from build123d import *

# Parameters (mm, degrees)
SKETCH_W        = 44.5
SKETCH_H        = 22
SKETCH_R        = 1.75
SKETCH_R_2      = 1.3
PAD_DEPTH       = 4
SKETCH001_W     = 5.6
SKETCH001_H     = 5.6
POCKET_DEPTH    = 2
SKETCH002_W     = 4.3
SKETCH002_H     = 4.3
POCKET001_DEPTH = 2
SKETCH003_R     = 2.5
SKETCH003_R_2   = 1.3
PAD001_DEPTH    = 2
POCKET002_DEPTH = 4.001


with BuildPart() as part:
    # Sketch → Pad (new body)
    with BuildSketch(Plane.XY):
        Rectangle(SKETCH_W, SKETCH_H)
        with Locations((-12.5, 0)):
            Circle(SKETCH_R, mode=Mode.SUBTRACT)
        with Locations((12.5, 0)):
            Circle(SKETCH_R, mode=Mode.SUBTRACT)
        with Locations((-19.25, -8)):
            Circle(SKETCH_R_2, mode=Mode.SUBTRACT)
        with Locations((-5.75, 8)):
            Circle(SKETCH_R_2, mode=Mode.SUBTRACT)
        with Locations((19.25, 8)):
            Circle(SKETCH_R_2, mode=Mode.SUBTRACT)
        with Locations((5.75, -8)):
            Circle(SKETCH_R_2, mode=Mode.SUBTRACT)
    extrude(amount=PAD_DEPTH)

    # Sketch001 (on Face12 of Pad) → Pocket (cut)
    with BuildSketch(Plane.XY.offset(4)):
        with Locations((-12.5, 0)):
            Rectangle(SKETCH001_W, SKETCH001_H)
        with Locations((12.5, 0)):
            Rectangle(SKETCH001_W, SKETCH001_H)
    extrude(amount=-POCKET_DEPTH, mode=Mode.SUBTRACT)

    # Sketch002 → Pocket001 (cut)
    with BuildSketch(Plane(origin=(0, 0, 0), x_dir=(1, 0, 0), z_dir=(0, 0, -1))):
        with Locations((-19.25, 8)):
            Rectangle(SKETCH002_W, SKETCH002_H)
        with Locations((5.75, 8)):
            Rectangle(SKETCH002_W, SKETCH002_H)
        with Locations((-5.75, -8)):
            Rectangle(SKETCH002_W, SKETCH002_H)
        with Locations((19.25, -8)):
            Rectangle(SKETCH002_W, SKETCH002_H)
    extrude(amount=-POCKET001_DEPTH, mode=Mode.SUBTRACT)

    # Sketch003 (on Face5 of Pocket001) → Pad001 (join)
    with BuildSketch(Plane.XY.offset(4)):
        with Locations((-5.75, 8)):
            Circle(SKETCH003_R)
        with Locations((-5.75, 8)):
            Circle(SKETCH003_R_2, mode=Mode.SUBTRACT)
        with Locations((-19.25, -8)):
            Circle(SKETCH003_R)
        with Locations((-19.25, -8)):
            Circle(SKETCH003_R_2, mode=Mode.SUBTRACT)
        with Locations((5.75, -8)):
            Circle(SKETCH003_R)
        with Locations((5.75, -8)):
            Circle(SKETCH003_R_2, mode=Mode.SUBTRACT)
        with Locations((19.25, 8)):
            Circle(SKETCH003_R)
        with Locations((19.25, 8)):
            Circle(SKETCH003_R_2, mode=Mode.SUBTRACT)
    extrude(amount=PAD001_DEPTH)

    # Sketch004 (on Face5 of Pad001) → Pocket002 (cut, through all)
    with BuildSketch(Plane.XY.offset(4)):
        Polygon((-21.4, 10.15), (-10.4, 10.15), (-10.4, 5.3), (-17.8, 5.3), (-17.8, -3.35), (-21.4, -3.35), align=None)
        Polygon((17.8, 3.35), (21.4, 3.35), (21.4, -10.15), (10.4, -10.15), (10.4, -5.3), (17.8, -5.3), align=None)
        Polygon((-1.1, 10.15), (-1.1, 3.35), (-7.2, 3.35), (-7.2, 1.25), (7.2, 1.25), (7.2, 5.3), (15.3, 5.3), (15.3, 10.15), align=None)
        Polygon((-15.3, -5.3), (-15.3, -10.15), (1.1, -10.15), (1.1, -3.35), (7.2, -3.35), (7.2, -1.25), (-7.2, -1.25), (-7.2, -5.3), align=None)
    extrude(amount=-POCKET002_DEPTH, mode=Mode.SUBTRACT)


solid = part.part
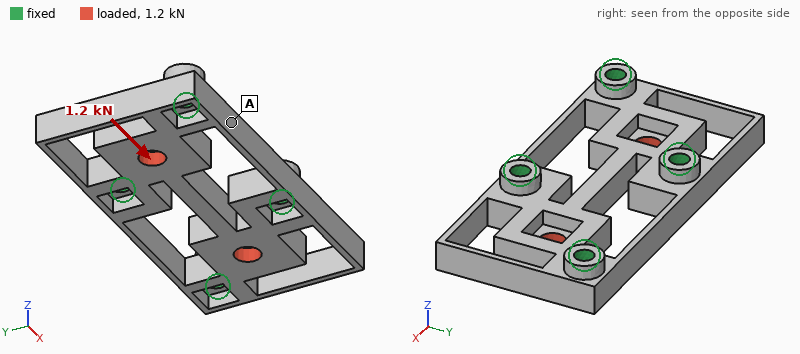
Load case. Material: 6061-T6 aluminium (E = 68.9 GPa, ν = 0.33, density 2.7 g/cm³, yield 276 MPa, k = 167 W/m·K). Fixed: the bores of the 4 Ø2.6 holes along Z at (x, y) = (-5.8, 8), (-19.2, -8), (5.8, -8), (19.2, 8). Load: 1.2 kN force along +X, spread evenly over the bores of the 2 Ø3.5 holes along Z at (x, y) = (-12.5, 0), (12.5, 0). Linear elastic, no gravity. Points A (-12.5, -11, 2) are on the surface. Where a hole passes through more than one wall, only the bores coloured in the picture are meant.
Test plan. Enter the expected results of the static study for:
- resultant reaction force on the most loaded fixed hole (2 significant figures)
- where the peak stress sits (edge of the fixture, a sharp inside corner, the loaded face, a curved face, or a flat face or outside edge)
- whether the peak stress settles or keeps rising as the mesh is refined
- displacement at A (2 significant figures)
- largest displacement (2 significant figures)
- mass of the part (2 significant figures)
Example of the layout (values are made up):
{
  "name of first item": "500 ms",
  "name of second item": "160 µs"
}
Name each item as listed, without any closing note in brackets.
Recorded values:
{
  "resultant reaction force on the most loaded fixed hole": "300 N",
  "where the peak stress sits": "edge of the fixture",
  "whether the peak stress settles or keeps rising as the mesh is refined": "keeps rising",
  "displacement at A": "3.2 µm",
  "largest displacement": "13 µm",
  "mass of the part": "5.4 g"
}
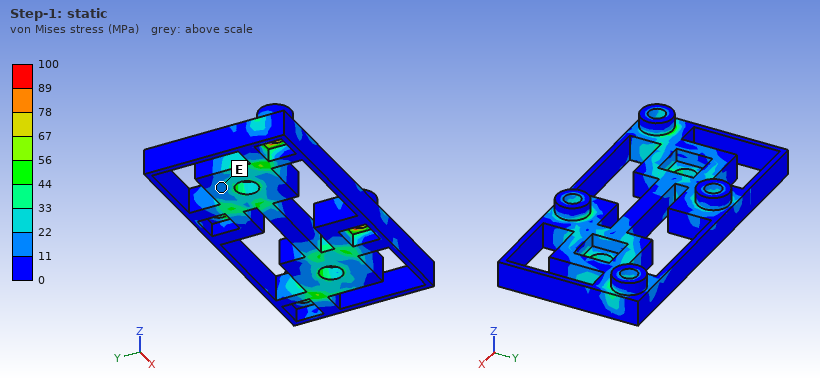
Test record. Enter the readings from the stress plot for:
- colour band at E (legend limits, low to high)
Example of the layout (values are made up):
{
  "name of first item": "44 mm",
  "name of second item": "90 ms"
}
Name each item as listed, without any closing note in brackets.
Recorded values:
{
  "colour band at E": "11 to 22 MPa"
}
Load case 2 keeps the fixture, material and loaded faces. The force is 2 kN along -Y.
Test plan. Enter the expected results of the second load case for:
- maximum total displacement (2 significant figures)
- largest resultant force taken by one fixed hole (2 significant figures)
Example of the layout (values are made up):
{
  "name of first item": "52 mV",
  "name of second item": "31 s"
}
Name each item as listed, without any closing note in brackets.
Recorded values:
{
  "maximum total displacement": "20 µm",
  "largest resultant force taken by one fixed hole": "530 N"
}
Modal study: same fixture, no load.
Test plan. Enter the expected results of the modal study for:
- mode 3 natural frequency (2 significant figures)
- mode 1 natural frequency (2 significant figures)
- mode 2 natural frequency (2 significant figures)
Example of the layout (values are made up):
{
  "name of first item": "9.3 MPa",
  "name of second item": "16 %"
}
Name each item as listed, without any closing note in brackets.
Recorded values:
{
  "mode 3 natural frequency": "15 kHz",
  "mode 1 natural frequency": "14 kHz",
  "mode 2 natural frequency": "14 kHz"
}
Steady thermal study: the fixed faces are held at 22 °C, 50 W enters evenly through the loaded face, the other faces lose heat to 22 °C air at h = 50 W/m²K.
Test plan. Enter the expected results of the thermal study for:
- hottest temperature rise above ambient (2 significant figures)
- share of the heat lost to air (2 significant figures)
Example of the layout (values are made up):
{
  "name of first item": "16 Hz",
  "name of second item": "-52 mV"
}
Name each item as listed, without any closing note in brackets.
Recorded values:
{
  "hottest temperature rise above ambient": "38 K",
  "share of the heat lost to air": "3.3 %"
}
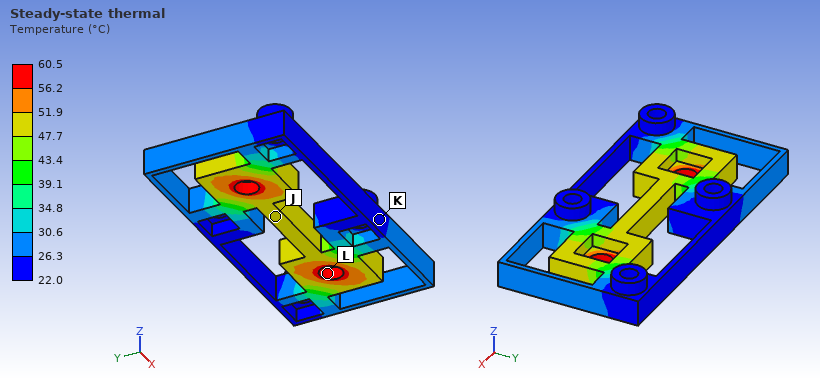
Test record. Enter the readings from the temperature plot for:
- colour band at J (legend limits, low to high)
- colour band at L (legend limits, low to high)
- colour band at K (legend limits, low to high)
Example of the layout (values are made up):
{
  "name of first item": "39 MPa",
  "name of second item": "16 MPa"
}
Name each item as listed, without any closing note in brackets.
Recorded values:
{
  "colour band at J": "47.7 to 51.9 °C",
  "colour band at L": "56.2 to 60.5 °C",
  "colour band at K": "22.0 to 26.3 °C"
}
